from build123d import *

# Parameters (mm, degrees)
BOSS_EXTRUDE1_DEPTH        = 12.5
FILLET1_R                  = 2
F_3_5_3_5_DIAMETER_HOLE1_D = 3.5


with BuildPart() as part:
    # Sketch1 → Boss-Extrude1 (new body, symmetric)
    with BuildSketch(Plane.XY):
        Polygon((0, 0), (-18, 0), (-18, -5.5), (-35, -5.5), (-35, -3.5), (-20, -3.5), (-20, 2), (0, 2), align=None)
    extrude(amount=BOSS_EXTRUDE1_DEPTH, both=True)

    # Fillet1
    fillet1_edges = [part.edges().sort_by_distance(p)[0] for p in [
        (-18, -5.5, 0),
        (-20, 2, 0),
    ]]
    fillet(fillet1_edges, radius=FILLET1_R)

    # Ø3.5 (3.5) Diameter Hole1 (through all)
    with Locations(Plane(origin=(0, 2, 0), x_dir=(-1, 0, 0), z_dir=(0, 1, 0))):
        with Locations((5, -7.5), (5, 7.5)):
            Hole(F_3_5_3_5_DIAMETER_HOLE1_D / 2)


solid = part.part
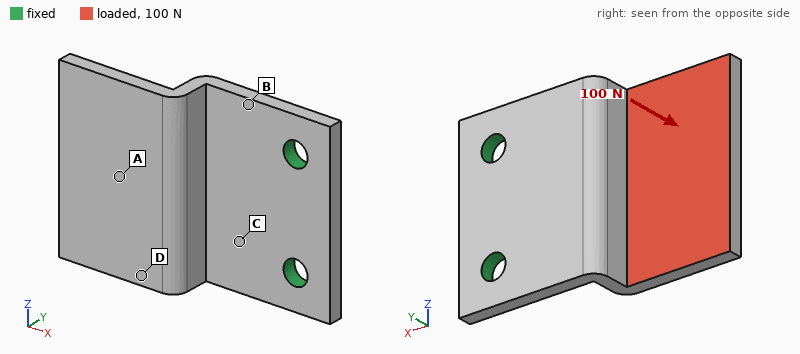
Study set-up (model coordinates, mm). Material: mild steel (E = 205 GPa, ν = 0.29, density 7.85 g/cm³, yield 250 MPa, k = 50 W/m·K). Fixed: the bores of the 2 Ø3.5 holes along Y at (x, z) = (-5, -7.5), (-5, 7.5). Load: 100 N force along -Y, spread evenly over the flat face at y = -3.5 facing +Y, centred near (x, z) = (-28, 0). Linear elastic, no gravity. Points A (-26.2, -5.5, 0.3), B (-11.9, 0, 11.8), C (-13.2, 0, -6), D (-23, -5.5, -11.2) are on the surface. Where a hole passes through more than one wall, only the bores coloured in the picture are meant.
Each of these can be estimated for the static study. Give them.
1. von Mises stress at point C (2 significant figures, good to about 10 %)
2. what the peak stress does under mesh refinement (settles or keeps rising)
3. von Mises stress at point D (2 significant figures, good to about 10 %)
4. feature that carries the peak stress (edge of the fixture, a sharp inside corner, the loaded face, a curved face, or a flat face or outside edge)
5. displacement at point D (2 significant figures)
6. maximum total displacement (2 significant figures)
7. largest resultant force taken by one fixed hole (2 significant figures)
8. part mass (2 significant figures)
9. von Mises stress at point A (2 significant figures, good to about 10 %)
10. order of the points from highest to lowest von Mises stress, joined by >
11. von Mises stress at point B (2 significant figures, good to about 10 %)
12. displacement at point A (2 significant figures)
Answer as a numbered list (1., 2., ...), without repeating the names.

1. 77 MPa
2. keeps rising
3. 29 MPa
4. edge of the fixture
5. 0.083 mm
6. 0.17 mm
7. 51 N
8. 15 g
9. 14 MPa
10. B > C > D > A
11. 97 MPa
12. 0.11 mm
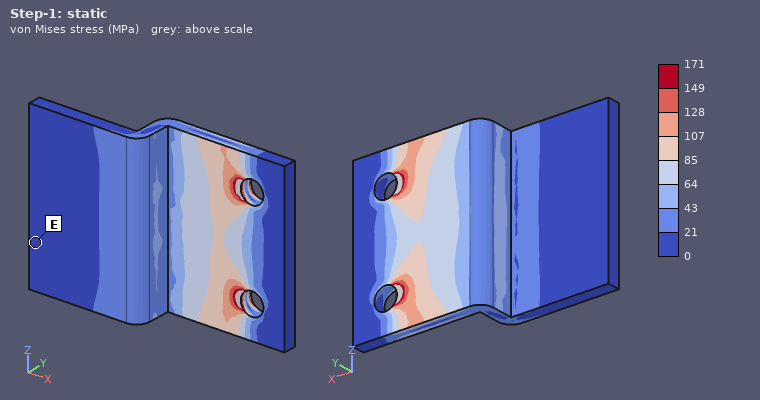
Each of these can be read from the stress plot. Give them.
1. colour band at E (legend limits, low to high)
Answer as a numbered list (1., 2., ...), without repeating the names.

1. 0 to 21 MPa
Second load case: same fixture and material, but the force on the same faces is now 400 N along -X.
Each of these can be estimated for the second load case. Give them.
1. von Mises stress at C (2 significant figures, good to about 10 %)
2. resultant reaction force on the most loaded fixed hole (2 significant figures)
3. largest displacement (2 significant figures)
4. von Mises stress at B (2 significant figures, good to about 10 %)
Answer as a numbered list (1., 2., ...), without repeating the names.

1. 110 MPa
2. 200 N
3. 0.16 mm
4. 120 MPa
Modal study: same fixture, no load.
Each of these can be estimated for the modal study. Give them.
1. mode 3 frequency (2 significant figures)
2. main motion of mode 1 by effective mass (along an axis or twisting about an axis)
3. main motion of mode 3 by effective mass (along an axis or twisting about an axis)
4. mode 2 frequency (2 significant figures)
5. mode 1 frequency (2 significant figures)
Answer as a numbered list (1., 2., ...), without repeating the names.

1. 8200 Hz
2. along Y
3. along Z
4. 5100 Hz
5. 1700 Hz
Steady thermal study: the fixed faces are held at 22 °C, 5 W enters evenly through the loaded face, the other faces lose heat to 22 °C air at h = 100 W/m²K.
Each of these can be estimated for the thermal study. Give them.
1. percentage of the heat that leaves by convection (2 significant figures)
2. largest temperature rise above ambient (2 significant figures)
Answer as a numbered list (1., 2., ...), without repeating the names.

1. 50 %
2. 32 K
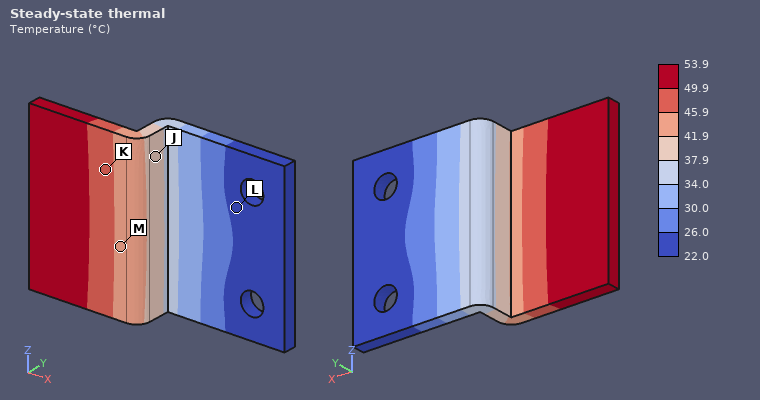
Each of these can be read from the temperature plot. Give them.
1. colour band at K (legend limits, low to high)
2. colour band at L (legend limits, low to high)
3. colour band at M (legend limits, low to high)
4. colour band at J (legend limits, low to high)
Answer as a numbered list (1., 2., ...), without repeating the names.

1. 45.9 to 49.9 °C
2. 22.0 to 26.0 °C
3. 41.9 to 45.9 °C
4. 37.9 to 41.9 °C
